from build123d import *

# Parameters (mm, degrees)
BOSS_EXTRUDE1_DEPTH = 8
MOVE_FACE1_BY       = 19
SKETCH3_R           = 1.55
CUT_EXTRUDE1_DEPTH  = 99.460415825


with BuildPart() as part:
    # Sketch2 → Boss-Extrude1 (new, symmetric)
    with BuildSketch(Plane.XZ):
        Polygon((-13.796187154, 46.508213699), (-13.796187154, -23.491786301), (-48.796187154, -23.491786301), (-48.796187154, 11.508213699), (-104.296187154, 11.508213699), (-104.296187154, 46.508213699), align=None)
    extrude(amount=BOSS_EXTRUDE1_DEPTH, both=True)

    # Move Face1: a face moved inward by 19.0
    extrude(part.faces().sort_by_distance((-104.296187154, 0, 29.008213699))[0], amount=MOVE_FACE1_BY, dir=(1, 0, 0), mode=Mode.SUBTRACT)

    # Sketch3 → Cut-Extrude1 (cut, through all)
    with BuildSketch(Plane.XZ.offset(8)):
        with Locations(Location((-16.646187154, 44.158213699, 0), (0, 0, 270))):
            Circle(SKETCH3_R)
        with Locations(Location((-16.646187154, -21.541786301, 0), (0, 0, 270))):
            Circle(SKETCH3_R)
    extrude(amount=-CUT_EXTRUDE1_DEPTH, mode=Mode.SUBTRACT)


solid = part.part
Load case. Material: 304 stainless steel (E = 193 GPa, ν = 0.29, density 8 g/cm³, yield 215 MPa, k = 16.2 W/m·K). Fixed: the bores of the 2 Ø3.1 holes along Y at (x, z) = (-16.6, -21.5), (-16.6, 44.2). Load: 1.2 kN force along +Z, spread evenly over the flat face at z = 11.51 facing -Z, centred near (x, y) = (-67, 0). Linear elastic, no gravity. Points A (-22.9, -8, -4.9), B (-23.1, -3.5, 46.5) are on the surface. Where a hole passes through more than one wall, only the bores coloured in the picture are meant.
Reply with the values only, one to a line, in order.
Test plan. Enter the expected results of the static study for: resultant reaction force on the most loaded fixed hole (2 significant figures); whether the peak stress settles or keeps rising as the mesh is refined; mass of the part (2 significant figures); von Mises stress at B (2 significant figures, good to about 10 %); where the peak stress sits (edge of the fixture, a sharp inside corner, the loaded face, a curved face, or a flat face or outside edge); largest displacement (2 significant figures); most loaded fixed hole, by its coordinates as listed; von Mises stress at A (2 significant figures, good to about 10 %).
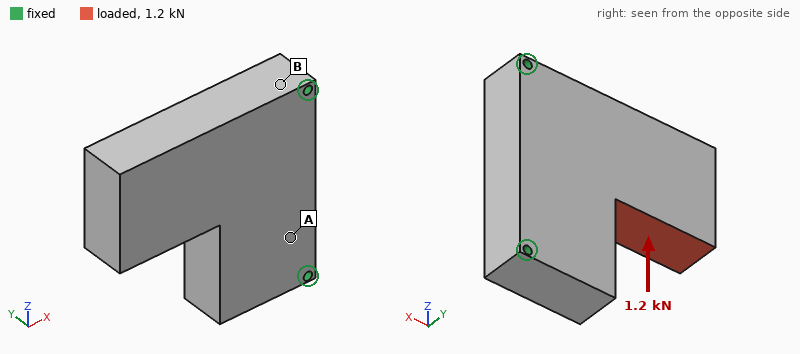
1.3 kN
keeps rising
480 g
8.4 MPa
edge of the fixture
5.2 µm
(-16.6, -21.5)
3.7 MPa
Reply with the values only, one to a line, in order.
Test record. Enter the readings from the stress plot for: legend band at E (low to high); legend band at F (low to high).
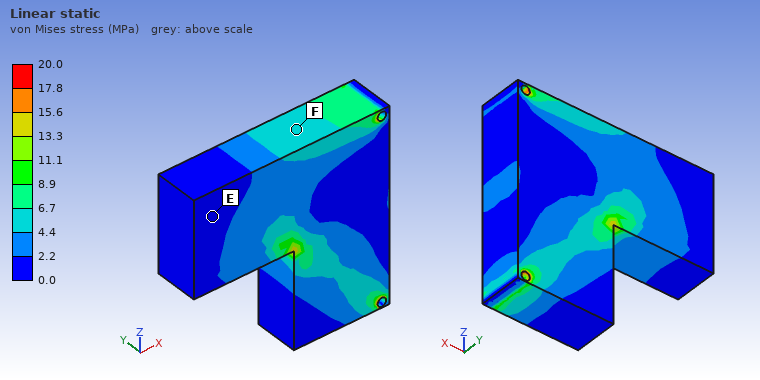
0.0 to 2.2 MPa
4.4 to 6.7 MPa
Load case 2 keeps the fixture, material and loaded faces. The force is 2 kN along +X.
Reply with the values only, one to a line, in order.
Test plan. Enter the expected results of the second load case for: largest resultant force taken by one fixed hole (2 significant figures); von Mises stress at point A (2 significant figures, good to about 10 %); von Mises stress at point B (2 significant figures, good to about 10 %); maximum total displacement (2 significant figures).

1.3 kN
4.1 MPa
4.5 MPa
6.1 µm
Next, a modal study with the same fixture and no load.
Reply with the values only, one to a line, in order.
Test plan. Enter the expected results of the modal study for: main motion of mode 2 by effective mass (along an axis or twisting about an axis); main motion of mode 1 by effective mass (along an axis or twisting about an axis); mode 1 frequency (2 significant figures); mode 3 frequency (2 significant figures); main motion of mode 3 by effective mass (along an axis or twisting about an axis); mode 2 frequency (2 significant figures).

along Z
along Y
2000 Hz
7600 Hz
along Y
6800 Hz
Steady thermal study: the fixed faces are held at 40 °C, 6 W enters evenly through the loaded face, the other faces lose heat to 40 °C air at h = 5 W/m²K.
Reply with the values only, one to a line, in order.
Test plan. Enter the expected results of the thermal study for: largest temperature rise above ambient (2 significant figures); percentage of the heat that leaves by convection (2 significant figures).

38 K
15 %
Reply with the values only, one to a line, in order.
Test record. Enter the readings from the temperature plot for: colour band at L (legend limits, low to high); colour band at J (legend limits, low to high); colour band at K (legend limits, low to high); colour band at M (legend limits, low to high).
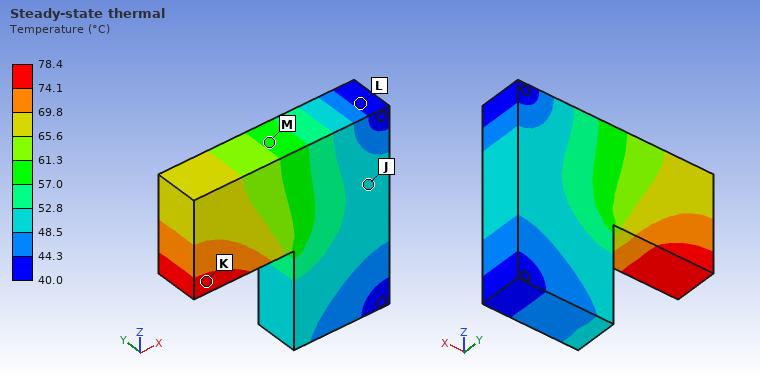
40.0 to 44.3 °C
48.5 to 52.8 °C
74.1 to 78.4 °C
57.0 to 61.3 °C
